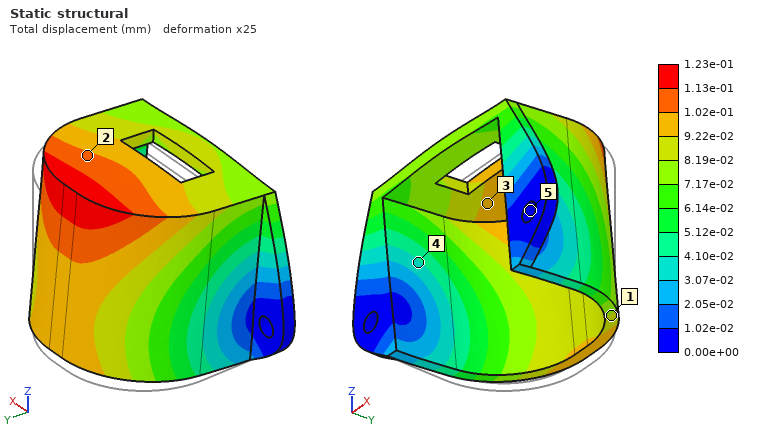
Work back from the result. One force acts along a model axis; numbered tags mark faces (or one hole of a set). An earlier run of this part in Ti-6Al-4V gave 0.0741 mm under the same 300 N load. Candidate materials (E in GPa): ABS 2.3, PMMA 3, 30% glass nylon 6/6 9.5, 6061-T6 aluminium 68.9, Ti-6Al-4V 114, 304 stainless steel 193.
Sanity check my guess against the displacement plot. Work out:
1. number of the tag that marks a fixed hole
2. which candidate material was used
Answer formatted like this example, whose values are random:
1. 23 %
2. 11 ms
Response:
1. 5
2. 6061-T6 aluminium
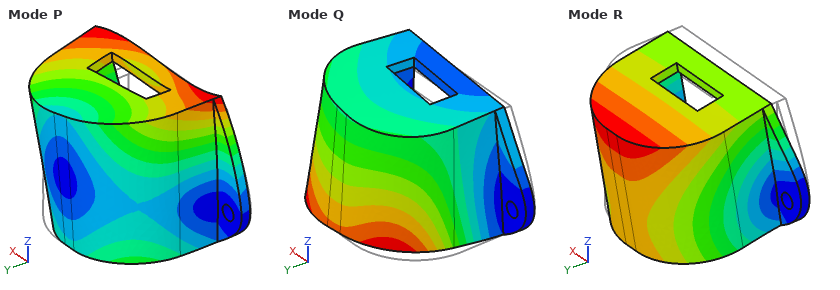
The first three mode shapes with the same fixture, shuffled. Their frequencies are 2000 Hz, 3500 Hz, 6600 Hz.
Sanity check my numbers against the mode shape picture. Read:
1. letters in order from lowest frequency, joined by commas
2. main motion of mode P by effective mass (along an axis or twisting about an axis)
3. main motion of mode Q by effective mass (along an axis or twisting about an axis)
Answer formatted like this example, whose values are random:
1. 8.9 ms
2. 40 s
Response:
1. R, Q, P
2. along X
3. along X
